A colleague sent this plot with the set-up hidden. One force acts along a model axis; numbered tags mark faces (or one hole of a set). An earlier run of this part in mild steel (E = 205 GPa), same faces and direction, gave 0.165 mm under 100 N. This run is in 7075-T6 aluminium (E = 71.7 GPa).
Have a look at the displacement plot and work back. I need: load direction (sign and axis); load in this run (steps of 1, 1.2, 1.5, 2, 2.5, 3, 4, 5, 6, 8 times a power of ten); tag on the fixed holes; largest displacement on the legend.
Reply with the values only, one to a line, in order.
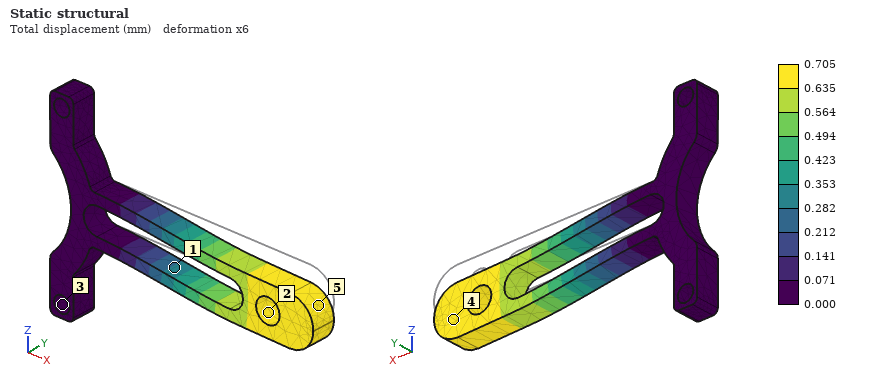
-Z
150 N
3
0.705 mm
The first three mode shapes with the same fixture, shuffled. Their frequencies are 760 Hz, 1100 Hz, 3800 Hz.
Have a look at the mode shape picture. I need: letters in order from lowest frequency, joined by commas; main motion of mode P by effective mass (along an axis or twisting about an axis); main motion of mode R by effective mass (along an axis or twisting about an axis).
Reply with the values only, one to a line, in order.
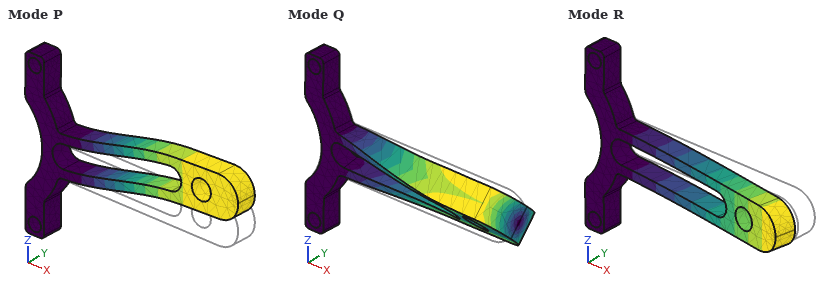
R, P, Q
along Z
along Y
